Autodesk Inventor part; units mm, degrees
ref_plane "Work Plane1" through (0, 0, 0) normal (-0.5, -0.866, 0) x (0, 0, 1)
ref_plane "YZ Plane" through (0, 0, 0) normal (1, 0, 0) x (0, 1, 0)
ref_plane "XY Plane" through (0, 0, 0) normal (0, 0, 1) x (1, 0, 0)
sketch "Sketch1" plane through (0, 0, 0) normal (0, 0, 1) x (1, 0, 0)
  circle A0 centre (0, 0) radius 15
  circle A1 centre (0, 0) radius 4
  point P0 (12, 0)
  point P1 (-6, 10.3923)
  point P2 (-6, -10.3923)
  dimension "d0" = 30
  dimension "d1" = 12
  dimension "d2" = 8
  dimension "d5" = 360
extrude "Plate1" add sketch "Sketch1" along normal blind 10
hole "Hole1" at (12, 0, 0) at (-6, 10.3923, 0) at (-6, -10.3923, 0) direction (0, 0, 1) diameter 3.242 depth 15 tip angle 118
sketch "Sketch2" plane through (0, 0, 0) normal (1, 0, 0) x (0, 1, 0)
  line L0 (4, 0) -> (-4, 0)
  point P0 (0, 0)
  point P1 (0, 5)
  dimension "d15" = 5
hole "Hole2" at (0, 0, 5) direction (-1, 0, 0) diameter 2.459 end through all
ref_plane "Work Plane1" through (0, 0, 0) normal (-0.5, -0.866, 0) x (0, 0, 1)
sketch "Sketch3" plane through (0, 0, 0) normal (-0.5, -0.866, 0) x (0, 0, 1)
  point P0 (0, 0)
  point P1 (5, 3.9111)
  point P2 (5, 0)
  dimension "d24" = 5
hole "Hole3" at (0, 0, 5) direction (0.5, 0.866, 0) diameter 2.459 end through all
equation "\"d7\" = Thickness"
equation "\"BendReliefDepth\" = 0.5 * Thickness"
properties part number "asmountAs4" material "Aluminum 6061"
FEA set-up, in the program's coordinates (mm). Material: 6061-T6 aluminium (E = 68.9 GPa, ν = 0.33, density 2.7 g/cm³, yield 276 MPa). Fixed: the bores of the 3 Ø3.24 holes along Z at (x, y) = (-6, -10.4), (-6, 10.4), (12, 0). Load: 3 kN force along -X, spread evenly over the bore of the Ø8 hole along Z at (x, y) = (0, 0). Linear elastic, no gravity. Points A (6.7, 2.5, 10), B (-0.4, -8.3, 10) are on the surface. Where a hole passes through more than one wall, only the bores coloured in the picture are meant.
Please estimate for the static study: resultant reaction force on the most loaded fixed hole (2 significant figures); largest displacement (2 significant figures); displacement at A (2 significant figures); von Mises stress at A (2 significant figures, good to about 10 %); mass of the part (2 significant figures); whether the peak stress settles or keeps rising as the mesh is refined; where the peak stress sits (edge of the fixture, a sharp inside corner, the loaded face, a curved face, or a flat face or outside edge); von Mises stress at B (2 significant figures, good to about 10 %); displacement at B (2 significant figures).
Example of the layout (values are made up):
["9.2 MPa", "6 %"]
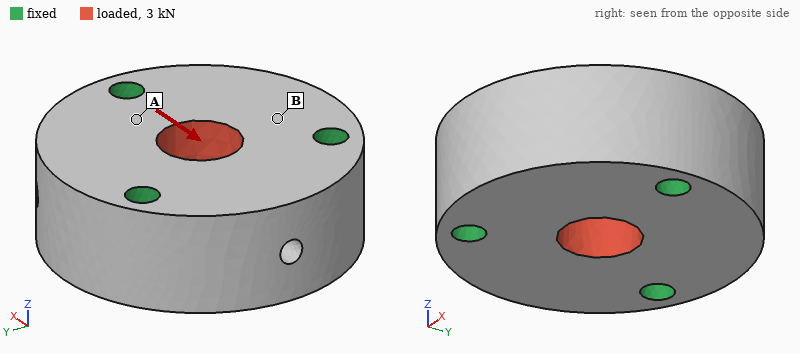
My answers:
["1.0 kN", "3.0 µm", "1.0 µm", "14 MPa", "17 g", "keeps rising", "edge of the fixture", "7.0 MPa", "0.94 µm"]
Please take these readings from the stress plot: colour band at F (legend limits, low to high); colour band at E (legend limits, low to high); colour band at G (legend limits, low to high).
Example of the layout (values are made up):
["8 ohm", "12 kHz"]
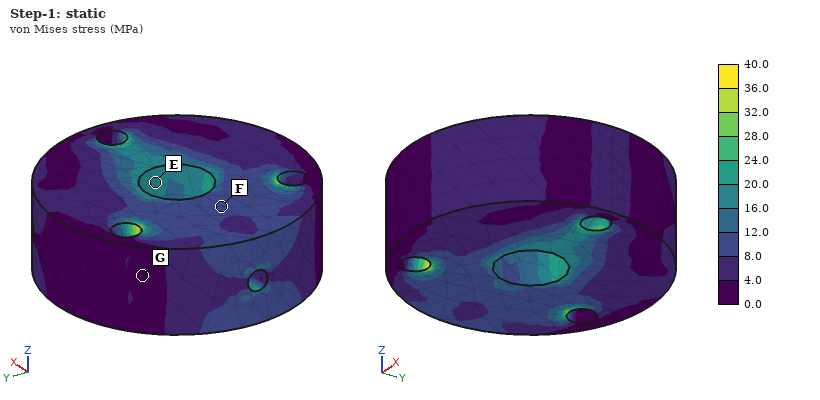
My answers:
["8.0 to 12.0 MPa", "16.0 to 20.0 MPa", "0.0 to 4.0 MPa"]
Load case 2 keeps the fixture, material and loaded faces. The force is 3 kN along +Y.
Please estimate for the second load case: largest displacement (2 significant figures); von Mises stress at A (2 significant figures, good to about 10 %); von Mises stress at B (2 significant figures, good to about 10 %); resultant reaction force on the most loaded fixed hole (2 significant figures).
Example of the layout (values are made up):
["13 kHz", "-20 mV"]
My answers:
["2.9 µm", "6.5 MPa", "11 MPa", "1.0 kN"]
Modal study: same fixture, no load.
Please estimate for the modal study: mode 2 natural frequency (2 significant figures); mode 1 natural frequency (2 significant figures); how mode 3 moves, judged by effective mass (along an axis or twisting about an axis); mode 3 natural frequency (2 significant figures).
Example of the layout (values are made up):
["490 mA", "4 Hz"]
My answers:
["49 kHz", "48 kHz", "along Z", "52 kHz"]
